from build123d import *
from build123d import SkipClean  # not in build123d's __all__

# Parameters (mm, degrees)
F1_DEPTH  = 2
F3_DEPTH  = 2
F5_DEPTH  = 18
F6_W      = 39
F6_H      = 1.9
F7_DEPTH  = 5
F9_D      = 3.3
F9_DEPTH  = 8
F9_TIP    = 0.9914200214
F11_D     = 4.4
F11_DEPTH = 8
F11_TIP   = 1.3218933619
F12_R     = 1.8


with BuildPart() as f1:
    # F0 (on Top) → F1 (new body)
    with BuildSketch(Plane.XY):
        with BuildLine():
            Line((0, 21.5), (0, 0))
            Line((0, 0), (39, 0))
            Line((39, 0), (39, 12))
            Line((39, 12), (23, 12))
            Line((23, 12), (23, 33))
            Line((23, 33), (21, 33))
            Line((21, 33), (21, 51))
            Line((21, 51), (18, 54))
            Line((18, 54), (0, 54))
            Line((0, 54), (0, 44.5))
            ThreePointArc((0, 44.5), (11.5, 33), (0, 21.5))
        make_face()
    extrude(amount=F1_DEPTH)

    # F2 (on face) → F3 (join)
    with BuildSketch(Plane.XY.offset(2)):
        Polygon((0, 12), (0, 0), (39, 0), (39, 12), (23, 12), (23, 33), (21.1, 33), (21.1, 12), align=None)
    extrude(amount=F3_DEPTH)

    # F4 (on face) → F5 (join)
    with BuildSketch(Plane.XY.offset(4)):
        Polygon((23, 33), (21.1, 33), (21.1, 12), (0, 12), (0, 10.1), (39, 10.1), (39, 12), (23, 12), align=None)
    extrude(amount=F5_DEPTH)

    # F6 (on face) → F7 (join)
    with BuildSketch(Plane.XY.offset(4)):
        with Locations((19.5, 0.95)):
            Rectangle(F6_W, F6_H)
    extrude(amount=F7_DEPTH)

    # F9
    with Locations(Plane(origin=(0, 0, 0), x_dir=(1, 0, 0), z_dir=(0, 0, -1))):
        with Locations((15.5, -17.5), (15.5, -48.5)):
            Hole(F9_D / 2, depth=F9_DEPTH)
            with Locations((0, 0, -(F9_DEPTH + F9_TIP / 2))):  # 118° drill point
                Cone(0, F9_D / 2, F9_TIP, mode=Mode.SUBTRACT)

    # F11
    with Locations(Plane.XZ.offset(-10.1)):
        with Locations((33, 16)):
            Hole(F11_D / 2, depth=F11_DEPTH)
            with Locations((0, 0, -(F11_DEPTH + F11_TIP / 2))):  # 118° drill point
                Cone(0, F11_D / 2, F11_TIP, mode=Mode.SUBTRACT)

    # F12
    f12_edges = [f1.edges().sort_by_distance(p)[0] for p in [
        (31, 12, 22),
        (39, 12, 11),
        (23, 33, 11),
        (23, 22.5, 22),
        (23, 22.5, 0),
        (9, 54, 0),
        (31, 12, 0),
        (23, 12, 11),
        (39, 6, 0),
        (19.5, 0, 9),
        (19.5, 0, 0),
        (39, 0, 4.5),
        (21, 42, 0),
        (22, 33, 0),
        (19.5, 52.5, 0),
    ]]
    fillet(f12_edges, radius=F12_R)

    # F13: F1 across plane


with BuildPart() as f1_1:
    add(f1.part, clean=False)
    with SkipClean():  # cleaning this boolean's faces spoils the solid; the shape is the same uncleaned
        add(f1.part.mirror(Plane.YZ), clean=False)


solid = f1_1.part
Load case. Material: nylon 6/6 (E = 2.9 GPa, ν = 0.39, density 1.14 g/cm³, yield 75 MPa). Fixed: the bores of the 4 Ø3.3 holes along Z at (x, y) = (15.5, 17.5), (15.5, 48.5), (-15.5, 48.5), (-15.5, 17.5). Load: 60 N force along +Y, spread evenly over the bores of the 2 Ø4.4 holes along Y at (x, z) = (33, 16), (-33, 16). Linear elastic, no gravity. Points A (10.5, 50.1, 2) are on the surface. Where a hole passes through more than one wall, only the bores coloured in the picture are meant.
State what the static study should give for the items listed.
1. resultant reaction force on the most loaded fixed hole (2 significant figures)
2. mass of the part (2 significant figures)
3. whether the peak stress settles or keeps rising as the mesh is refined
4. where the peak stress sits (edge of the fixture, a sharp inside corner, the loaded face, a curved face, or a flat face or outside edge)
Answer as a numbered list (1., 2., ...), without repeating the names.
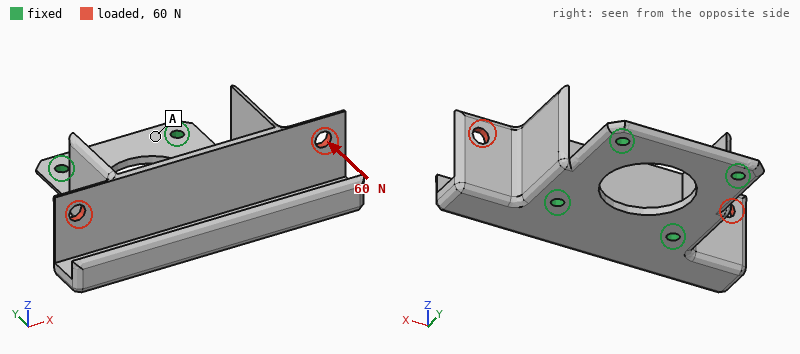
1. 25 N
2. 13 g
3. keeps rising
4. a sharp inside corner
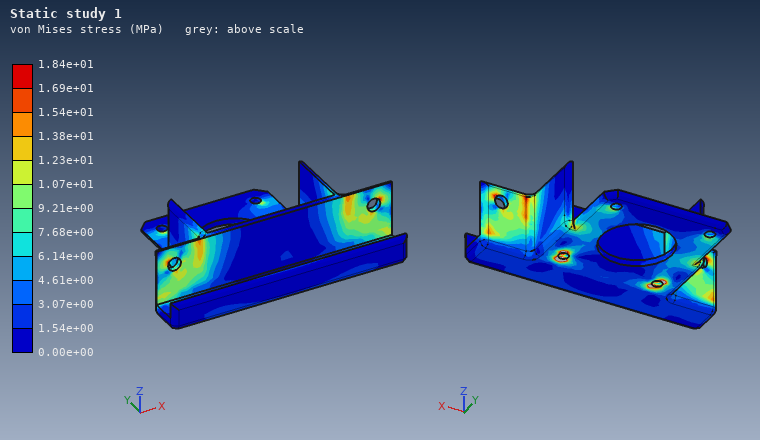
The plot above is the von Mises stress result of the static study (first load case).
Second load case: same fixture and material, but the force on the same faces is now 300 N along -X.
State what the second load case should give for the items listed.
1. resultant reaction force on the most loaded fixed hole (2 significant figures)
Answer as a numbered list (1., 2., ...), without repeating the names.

1. 210 N
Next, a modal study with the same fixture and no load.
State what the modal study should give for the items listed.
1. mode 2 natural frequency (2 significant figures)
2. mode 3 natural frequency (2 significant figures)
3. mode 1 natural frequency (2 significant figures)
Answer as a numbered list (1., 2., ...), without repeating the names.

1. 1100 Hz
2. 1700 Hz
3. 880 Hz
